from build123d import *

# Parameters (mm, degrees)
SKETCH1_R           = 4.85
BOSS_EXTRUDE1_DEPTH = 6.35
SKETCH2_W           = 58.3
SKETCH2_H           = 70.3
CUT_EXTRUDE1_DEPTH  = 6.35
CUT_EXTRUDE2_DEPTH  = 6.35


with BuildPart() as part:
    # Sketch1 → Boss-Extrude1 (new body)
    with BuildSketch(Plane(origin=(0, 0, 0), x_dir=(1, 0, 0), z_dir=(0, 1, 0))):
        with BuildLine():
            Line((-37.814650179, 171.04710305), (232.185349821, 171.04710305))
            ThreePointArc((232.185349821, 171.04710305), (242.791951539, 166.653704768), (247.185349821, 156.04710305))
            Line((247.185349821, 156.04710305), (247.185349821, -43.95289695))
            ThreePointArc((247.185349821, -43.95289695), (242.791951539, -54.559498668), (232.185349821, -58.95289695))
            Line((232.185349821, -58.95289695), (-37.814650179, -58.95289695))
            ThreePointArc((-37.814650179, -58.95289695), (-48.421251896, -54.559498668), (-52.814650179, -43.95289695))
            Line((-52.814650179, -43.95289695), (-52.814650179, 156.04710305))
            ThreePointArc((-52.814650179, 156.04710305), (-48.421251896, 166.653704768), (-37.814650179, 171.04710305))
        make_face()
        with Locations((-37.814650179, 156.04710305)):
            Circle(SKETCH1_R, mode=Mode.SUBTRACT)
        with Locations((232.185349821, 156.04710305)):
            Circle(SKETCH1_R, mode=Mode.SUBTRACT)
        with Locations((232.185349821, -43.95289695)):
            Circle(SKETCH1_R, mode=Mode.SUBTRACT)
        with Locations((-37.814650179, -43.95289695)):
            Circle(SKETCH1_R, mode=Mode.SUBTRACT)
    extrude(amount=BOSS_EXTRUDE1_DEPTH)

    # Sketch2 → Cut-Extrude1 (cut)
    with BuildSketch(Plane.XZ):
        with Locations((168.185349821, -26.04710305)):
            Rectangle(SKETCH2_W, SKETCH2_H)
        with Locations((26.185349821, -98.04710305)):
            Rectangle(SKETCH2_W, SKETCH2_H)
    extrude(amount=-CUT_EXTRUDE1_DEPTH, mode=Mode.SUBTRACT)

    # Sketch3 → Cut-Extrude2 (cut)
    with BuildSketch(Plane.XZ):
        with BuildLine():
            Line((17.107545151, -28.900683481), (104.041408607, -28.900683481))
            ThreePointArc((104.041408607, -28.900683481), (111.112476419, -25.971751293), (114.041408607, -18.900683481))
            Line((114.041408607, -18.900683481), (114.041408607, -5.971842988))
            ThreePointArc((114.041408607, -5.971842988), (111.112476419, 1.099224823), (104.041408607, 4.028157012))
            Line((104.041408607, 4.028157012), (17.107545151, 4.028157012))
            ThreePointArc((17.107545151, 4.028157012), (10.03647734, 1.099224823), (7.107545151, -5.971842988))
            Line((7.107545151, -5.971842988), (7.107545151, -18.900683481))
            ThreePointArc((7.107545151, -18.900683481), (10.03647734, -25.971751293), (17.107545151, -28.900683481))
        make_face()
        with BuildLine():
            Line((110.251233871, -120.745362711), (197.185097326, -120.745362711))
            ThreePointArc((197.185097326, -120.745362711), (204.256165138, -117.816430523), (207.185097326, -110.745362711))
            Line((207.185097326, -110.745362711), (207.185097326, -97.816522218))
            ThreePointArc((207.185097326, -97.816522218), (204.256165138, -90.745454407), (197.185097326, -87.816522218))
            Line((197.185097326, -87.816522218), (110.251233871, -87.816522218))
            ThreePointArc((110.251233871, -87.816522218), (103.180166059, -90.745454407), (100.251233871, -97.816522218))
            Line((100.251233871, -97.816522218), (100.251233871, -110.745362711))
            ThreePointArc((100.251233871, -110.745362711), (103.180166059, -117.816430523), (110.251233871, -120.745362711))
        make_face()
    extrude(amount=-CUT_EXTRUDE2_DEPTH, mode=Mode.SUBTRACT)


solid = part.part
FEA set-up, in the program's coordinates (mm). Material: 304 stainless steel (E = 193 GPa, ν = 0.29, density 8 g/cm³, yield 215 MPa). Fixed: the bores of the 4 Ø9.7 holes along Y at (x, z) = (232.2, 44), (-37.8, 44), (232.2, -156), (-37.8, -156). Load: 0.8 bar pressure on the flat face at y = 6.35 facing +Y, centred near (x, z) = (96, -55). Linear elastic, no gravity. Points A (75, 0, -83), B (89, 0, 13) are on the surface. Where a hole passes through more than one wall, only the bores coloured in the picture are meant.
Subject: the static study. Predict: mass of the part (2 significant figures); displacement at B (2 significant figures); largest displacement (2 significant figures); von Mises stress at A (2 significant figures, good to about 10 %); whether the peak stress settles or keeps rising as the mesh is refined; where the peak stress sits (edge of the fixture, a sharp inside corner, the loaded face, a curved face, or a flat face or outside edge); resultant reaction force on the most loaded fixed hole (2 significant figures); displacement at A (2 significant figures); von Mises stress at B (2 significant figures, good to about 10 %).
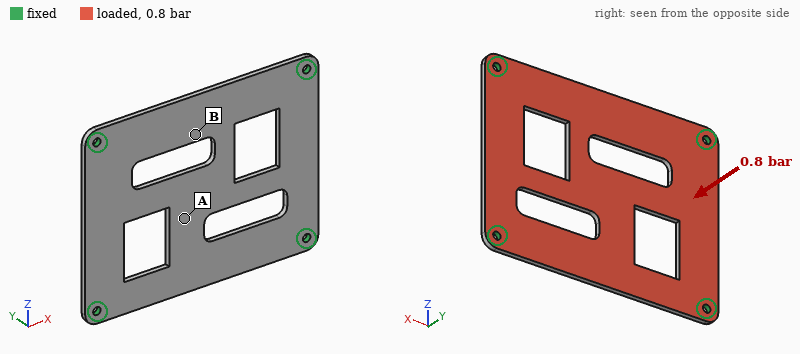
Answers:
2.7 kg
0.41 mm
0.49 mm
22 MPa
keeps rising
edge of the fixture
1.1 kN
0.46 mm
44 MPa
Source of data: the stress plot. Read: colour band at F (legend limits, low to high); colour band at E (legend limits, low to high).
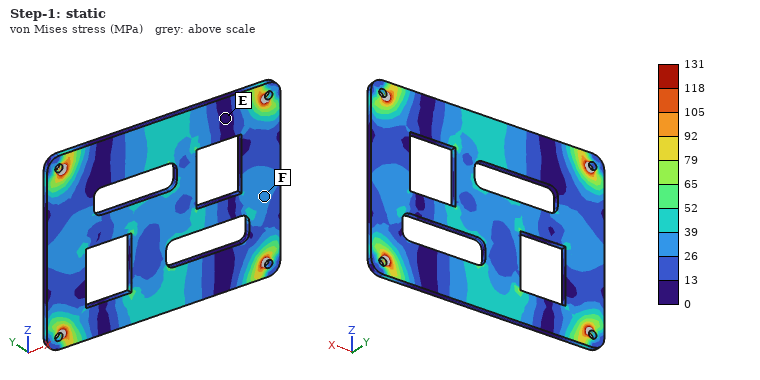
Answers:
26 to 39 MPa
0 to 13 MPa
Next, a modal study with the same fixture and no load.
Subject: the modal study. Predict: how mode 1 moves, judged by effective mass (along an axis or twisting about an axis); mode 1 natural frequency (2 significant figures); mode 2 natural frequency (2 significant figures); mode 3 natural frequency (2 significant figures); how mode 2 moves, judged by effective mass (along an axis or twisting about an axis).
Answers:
along Y
340 Hz
510 Hz
690 Hz
twisting about X
